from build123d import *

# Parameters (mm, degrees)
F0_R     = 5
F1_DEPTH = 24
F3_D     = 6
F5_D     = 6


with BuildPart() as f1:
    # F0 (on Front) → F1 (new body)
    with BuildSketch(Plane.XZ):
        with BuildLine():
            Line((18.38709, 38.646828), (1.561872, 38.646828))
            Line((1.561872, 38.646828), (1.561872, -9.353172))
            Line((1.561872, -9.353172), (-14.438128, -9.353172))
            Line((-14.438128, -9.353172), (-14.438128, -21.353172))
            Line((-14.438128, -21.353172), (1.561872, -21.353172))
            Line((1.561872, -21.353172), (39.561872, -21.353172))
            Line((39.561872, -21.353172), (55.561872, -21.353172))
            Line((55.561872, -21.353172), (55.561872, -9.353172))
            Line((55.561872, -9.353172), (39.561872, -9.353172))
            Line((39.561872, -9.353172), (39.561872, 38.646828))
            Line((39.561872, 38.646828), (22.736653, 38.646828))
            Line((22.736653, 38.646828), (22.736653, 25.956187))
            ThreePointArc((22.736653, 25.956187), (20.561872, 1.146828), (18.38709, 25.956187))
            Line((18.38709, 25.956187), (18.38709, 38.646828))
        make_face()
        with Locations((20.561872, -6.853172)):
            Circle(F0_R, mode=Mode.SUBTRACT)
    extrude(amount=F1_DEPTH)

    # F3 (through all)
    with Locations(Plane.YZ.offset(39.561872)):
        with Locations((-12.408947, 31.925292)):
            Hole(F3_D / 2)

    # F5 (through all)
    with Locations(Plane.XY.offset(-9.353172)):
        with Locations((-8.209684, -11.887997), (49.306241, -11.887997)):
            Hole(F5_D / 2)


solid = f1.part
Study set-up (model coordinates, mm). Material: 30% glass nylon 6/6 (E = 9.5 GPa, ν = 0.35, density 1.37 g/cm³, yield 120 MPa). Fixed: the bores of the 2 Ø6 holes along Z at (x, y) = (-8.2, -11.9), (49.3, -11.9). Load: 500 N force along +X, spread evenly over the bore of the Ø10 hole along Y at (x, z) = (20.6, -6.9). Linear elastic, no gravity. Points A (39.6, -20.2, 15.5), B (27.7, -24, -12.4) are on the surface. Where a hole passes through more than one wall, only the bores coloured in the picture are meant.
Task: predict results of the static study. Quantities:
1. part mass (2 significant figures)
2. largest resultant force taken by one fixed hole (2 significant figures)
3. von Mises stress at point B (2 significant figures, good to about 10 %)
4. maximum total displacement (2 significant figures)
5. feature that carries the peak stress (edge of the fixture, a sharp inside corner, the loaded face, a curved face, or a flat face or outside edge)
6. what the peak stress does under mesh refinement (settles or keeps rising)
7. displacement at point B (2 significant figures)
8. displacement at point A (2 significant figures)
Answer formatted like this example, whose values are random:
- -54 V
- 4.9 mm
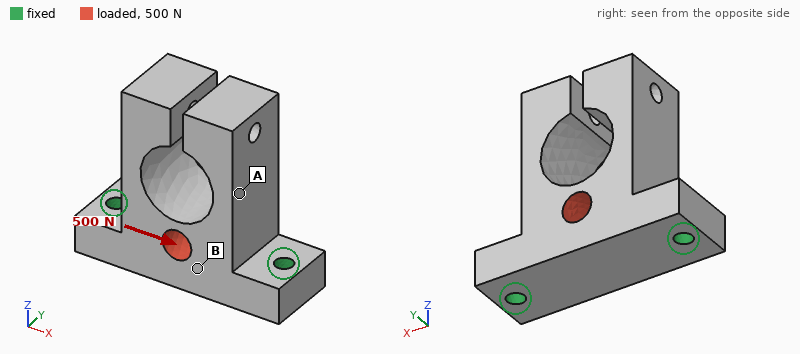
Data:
- 65 g
- 260 N
- 0.67 MPa
- 9.6 µm
- edge of the fixture
- keeps rising
- 2.2 µm
- 6.4 µm
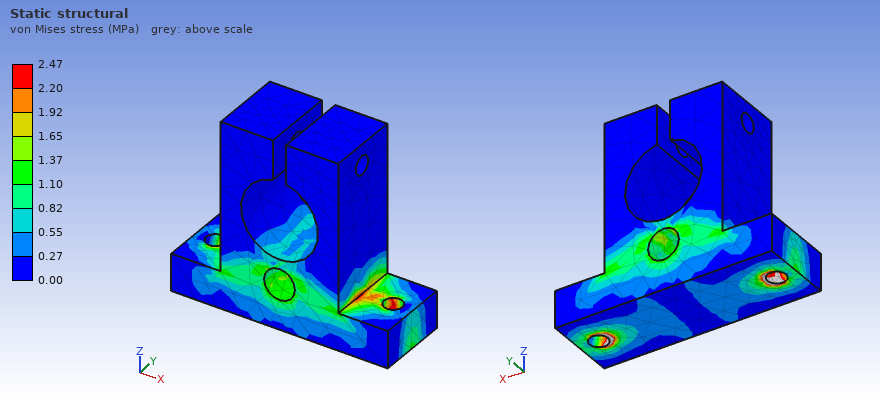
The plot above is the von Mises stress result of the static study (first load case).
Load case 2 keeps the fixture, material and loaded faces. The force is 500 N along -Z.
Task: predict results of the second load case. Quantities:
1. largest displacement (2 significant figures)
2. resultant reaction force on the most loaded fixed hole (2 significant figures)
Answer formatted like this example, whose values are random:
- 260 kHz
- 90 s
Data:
- 15 µm
- 270 N
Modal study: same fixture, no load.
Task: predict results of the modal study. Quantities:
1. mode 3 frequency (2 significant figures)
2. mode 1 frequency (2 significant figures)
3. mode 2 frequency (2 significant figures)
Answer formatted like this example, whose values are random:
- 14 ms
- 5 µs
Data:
- 1500 Hz
- 1500 Hz
- 1500 Hz
